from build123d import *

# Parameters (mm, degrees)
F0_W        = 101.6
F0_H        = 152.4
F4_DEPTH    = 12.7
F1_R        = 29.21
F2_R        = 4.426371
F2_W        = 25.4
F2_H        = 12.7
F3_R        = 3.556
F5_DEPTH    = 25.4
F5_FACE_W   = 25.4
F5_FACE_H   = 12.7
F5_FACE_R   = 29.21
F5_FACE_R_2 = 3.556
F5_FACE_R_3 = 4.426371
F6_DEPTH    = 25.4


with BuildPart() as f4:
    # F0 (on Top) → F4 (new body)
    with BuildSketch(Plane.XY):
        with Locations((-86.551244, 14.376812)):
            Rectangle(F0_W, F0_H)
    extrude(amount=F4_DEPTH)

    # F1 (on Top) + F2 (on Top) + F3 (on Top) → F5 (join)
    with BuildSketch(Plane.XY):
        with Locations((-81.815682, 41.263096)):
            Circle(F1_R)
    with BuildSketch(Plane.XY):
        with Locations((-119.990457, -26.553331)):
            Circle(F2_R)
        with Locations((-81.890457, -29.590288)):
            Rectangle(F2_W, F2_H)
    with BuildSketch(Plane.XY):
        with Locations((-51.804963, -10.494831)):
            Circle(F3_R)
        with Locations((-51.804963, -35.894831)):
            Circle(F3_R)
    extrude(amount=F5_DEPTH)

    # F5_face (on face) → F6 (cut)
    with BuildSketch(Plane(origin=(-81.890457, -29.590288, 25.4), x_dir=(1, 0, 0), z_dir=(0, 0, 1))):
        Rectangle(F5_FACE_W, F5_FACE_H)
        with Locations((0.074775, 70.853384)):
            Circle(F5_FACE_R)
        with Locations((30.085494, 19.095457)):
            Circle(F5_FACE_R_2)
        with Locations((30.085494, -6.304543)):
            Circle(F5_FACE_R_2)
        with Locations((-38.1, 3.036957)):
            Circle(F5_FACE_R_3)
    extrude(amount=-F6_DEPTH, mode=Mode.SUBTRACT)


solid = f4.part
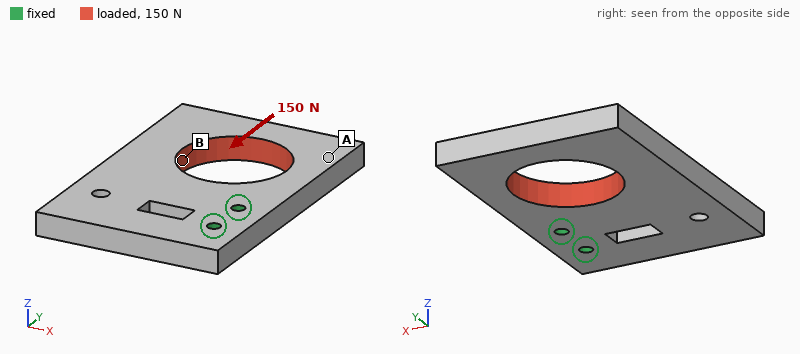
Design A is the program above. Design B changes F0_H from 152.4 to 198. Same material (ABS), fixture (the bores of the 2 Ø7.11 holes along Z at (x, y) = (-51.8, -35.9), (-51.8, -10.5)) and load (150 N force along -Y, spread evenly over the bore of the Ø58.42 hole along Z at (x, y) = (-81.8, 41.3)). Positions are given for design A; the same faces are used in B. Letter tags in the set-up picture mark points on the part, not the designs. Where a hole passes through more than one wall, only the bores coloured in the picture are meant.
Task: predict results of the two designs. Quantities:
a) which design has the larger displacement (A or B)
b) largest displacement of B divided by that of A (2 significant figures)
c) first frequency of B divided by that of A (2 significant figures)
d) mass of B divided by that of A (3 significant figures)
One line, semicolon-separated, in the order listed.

B; 1.1; 0.69; 1.38
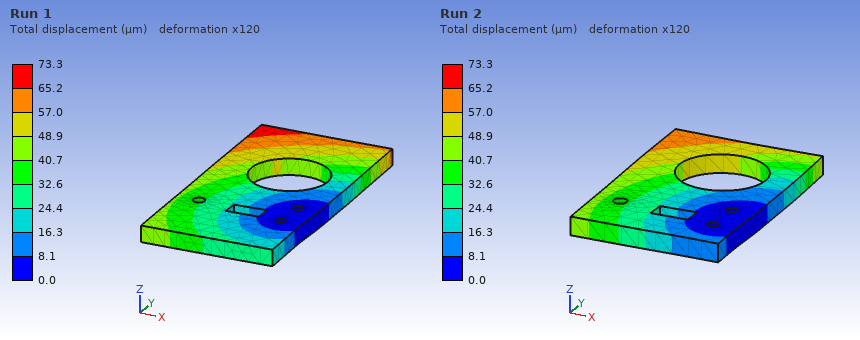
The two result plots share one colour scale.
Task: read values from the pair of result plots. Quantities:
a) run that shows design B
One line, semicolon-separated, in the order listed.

Run 1
